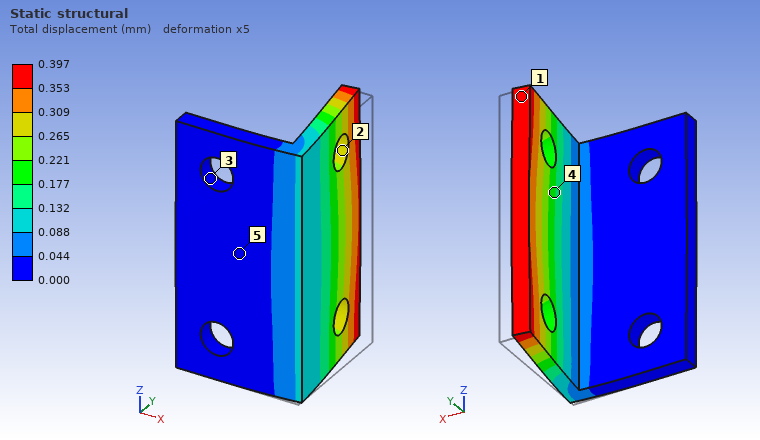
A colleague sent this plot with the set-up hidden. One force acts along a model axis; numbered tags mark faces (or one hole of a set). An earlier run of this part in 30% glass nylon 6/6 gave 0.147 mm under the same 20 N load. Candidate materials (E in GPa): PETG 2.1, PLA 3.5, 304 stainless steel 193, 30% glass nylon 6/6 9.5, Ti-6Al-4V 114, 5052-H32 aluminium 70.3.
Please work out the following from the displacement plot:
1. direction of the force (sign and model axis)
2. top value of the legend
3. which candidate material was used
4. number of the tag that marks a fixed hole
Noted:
-X
0.397 mm
PLA
3
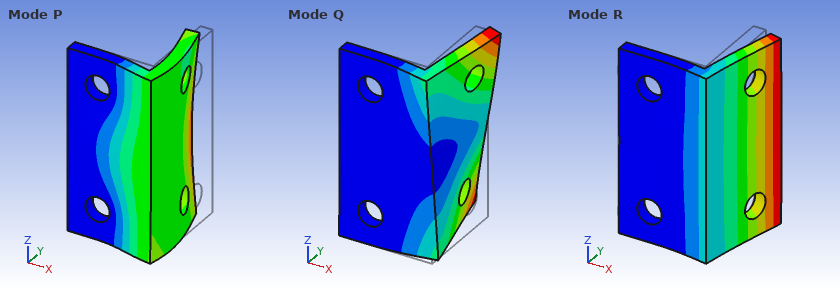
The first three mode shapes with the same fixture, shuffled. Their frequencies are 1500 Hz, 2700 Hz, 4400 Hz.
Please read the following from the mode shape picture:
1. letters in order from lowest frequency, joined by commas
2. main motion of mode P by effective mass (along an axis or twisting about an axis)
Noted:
R, Q, P
along Y
